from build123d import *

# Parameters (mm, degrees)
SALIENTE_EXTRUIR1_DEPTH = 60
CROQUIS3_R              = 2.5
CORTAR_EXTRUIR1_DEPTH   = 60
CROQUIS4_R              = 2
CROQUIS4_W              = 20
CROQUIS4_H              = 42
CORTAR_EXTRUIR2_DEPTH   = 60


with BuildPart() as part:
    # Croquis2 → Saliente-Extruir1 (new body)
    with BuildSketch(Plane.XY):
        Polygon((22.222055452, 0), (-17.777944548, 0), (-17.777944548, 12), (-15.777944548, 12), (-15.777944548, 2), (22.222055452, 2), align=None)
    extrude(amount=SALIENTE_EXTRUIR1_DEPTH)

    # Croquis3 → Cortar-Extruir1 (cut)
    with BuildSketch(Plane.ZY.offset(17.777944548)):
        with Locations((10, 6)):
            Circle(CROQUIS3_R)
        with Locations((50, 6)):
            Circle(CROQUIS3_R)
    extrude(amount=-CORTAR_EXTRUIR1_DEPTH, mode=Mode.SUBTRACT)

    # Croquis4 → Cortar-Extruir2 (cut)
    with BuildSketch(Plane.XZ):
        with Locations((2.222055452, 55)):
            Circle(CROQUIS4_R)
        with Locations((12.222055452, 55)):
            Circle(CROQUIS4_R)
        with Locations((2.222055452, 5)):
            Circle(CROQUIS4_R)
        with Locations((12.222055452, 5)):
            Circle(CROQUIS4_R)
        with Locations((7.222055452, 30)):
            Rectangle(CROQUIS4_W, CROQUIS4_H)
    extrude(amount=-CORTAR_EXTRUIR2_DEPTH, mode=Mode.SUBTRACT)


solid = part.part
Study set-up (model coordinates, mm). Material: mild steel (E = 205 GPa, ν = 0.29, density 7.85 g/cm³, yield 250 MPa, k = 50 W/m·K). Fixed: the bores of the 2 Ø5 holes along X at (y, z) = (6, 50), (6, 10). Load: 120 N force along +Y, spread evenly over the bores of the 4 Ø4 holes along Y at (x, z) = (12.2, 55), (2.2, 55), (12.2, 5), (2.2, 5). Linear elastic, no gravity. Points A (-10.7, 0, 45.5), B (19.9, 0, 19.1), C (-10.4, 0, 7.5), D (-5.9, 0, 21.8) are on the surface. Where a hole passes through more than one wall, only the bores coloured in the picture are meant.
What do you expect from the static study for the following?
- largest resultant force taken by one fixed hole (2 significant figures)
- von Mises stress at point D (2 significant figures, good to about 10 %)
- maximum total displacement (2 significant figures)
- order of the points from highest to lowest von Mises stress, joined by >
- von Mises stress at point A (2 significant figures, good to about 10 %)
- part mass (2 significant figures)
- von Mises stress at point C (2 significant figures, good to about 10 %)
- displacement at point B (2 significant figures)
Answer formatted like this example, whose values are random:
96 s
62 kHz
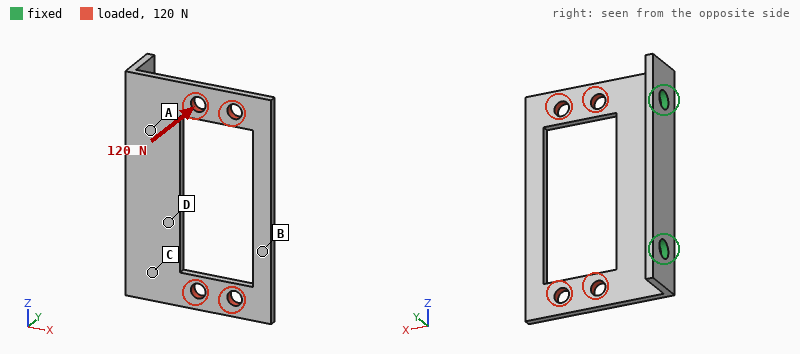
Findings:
60 N
33 MPa
0.34 mm
C > A > D > B
56 MPa
33 g
79 MPa
0.30 mm
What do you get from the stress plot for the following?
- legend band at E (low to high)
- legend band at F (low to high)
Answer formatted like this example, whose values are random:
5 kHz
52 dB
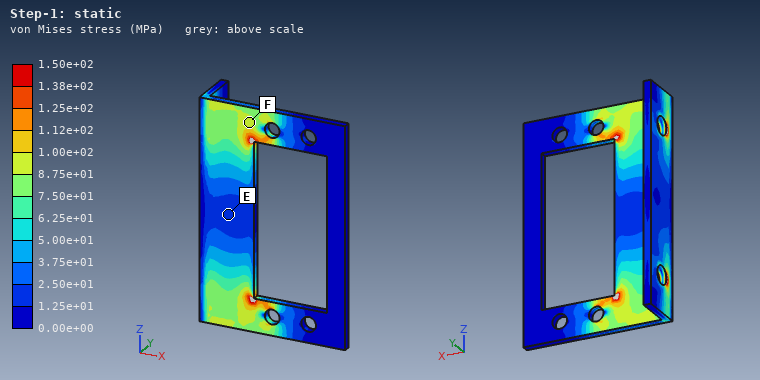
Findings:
1.25e+01 to 2.50e+01 MPa
8.75e+01 to 1.00e+02 MPa
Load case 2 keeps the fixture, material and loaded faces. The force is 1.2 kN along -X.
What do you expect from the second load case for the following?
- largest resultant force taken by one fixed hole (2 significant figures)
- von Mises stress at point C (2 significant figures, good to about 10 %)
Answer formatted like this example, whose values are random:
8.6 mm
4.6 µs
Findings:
620 N
39 MPa
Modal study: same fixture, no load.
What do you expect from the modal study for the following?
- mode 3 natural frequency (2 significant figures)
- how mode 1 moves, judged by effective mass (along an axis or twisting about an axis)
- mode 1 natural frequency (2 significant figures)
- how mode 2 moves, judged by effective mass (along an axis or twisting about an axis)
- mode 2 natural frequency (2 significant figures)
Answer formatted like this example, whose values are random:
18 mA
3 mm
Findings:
3300 Hz
along Y
860 Hz
twisting about X
1500 Hz
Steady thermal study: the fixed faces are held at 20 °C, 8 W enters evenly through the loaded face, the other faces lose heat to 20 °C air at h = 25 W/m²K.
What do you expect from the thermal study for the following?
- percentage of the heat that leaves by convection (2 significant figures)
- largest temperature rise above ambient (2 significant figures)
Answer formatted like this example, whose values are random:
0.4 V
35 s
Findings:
37 %
68 K
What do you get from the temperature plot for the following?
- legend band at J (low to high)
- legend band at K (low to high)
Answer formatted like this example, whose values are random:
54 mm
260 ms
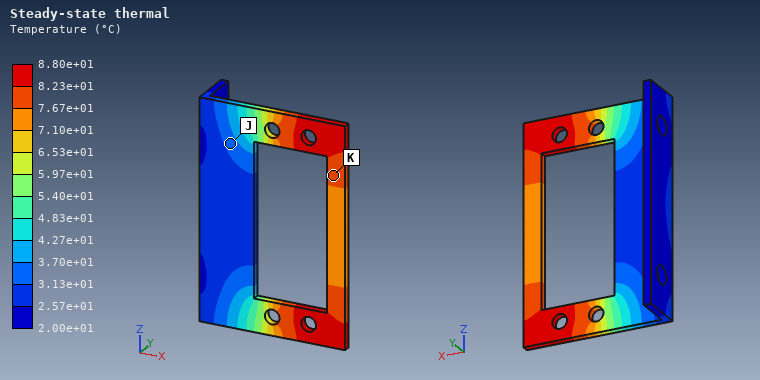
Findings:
3.13e+01 to 3.70e+01 °C
7.67e+01 to 8.23e+01 °C
